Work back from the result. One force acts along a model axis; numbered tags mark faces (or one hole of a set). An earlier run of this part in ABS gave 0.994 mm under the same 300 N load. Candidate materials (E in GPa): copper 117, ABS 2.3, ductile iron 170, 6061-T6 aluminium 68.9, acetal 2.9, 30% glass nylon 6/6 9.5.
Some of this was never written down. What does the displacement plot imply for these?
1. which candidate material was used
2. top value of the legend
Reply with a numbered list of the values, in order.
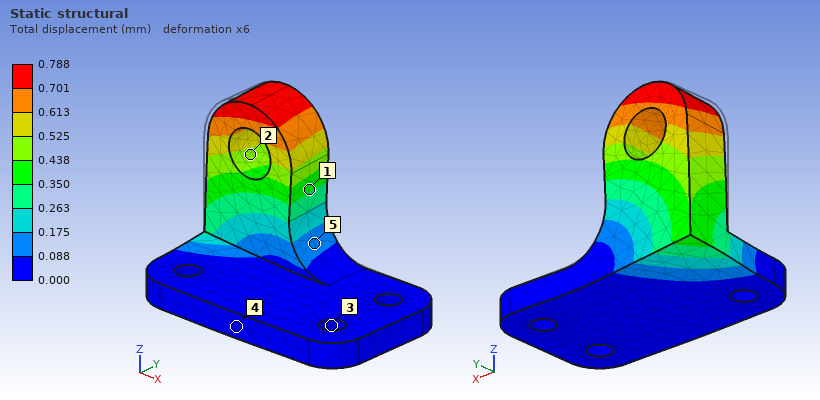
1. acetal
2. 0.788 mm
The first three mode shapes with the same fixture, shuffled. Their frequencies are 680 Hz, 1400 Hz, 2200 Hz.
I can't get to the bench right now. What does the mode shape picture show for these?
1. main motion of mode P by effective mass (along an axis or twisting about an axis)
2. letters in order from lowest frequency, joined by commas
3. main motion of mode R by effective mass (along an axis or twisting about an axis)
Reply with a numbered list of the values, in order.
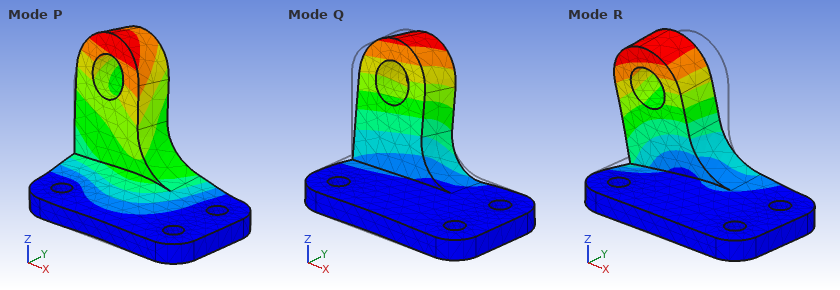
1. along Z
2. Q, R, P
3. along X
